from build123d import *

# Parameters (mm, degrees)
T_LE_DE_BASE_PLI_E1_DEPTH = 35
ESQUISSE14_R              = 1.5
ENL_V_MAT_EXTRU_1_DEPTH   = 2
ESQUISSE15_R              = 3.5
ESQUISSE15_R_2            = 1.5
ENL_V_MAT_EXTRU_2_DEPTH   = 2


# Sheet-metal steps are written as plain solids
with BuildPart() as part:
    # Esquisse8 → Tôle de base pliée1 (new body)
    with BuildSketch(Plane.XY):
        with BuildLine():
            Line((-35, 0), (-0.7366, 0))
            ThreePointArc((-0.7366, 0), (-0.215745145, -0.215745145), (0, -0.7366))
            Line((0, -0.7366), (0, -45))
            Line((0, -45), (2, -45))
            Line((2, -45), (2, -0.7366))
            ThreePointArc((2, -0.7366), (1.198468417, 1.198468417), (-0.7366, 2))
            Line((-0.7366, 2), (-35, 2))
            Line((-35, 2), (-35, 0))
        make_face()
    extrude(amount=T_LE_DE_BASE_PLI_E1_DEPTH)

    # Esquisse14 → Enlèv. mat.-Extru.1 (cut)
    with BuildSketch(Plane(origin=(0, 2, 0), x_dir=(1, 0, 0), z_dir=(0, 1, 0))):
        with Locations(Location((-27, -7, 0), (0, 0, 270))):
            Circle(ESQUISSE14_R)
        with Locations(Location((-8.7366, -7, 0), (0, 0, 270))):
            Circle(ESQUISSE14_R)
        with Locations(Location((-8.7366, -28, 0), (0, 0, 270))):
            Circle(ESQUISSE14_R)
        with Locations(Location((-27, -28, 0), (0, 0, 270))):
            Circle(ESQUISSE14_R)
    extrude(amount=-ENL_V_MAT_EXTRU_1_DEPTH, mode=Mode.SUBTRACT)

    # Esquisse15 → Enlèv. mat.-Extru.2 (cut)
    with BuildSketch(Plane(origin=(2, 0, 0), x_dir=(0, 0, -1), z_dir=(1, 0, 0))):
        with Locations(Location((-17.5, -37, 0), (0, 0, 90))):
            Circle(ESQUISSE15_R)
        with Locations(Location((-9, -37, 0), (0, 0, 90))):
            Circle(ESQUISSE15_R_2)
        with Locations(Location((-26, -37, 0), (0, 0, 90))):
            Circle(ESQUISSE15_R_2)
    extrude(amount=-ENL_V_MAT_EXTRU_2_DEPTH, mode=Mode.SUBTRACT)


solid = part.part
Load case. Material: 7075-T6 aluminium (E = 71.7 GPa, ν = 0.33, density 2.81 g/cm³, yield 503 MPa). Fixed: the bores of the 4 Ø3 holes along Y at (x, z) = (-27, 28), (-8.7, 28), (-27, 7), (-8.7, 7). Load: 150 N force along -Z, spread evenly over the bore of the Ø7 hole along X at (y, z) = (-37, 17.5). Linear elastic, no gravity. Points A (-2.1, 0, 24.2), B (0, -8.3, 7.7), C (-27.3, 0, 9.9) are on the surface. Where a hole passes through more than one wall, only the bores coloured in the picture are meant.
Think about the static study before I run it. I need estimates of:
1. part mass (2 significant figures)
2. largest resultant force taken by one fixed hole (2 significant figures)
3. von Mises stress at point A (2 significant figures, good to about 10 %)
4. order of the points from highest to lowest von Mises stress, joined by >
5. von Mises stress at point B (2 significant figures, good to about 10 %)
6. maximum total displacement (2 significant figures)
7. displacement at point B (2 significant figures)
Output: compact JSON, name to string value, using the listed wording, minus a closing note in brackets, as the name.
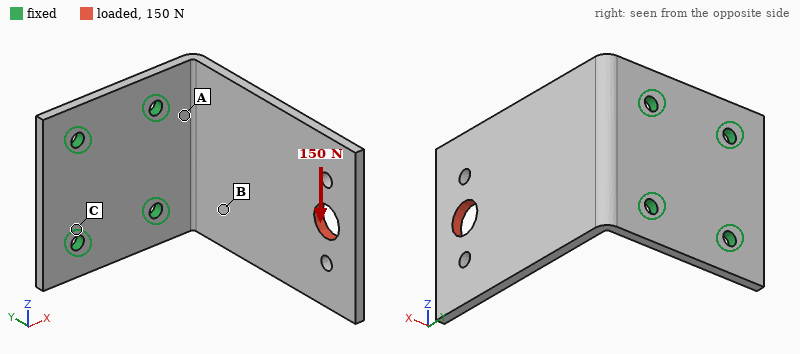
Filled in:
{"part mass": "16 g", "largest resultant force taken by one fixed hole": "270 N", "von Mises stress at point A": "69 MPa", "order of the points from highest to lowest von Mises stress, joined by >": "A > B > C", "von Mises stress at point B": "32 MPa", "maximum total displacement": "0.26 mm", "displacement at point B": "0.074 mm"}
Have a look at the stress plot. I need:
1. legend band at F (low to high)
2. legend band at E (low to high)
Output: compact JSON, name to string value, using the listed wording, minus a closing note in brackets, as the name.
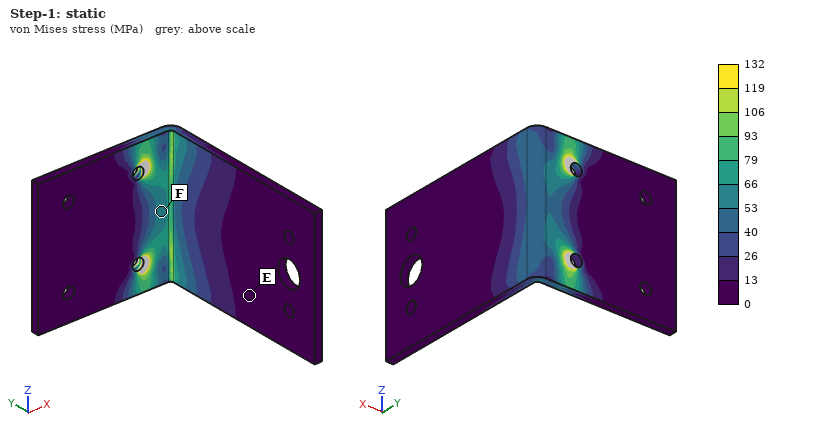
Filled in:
{"legend band at F": "53 to 66 MPa", "legend band at E": "0 to 13 MPa"}
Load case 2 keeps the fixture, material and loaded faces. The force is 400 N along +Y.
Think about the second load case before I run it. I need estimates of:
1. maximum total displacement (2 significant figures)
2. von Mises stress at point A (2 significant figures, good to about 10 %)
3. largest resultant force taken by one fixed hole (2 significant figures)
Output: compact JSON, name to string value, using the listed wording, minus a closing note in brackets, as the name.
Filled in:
{"maximum total displacement": "0.50 mm", "von Mises stress at point A": "52 MPa", "largest resultant force taken by one fixed hole": "220 N"}
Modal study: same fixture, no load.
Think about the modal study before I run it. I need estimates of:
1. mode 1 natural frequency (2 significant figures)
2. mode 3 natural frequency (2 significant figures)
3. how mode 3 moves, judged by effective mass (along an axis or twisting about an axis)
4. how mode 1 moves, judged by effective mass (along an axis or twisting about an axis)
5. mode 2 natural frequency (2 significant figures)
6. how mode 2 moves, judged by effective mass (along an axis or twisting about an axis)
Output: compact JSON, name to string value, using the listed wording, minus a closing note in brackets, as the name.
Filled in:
{"mode 1 natural frequency": "620 Hz", "mode 3 natural frequency": "2500 Hz", "how mode 3 moves, judged by effective mass": "along Z", "how mode 1 moves, judged by effective mass": "along X", "mode 2 natural frequency": "1800 Hz", "how mode 2 moves, judged by effective mass": "along Z"}
